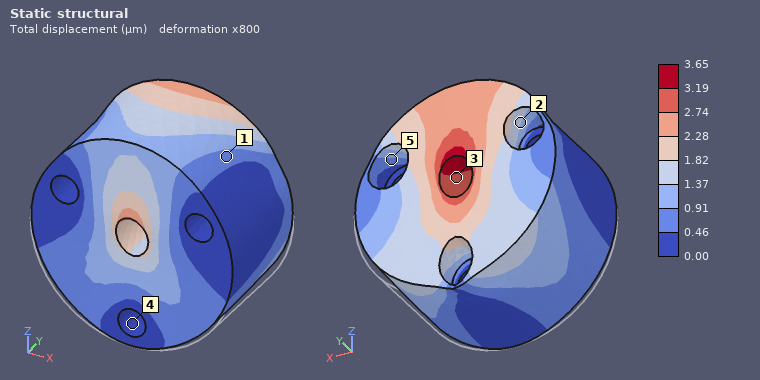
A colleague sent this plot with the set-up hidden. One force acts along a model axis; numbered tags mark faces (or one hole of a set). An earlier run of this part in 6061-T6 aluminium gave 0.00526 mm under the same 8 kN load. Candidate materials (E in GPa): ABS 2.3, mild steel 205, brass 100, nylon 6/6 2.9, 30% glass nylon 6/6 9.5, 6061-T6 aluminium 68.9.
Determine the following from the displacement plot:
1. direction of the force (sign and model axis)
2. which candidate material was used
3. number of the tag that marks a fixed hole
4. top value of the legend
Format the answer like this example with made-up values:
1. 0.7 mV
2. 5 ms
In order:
1. +Z
2. brass
3. 4
4. 3.65 µm
